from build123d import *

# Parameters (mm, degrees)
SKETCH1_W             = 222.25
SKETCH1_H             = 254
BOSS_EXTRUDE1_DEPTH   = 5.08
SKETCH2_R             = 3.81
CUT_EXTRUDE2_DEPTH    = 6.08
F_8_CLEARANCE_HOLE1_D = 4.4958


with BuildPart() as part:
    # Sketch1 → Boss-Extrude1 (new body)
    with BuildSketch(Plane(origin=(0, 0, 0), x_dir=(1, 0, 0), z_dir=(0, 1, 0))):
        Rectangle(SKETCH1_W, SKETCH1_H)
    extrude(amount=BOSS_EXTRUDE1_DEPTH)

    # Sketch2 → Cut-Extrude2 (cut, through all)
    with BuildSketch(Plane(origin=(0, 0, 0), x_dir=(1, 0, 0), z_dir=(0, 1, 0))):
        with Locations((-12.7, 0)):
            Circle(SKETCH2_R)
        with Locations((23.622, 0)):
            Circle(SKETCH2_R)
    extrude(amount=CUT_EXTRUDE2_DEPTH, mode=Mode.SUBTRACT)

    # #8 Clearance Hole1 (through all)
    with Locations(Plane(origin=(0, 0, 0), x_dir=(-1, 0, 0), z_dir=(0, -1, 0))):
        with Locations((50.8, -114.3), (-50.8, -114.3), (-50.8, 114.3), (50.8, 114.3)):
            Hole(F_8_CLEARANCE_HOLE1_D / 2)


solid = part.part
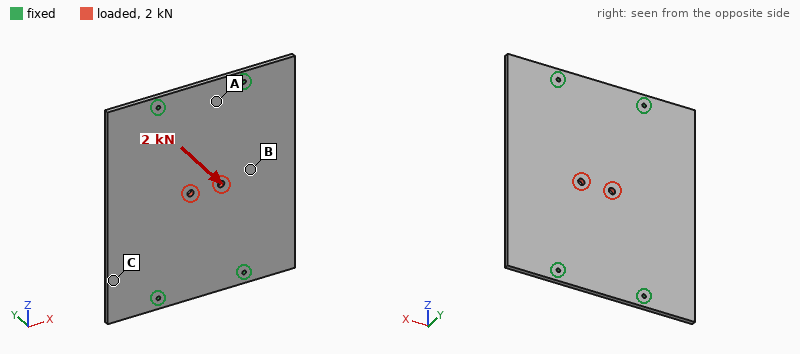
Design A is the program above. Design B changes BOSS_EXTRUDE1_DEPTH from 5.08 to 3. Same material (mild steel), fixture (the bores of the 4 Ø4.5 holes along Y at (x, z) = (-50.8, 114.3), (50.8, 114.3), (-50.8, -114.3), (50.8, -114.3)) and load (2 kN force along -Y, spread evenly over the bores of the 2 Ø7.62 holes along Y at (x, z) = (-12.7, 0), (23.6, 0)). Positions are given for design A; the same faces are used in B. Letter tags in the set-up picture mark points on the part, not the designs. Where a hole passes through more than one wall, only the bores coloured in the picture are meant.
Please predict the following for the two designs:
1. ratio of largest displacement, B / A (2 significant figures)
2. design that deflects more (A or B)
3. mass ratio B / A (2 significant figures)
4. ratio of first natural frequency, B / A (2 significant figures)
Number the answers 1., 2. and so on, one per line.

1. 4.7
2. B
3. 0.59
4. 0.61
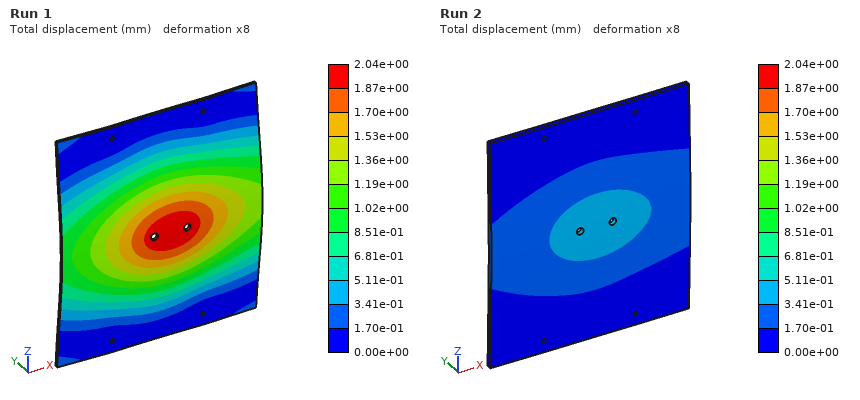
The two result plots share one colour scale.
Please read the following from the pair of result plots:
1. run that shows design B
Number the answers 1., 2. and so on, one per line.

1. Run 1
